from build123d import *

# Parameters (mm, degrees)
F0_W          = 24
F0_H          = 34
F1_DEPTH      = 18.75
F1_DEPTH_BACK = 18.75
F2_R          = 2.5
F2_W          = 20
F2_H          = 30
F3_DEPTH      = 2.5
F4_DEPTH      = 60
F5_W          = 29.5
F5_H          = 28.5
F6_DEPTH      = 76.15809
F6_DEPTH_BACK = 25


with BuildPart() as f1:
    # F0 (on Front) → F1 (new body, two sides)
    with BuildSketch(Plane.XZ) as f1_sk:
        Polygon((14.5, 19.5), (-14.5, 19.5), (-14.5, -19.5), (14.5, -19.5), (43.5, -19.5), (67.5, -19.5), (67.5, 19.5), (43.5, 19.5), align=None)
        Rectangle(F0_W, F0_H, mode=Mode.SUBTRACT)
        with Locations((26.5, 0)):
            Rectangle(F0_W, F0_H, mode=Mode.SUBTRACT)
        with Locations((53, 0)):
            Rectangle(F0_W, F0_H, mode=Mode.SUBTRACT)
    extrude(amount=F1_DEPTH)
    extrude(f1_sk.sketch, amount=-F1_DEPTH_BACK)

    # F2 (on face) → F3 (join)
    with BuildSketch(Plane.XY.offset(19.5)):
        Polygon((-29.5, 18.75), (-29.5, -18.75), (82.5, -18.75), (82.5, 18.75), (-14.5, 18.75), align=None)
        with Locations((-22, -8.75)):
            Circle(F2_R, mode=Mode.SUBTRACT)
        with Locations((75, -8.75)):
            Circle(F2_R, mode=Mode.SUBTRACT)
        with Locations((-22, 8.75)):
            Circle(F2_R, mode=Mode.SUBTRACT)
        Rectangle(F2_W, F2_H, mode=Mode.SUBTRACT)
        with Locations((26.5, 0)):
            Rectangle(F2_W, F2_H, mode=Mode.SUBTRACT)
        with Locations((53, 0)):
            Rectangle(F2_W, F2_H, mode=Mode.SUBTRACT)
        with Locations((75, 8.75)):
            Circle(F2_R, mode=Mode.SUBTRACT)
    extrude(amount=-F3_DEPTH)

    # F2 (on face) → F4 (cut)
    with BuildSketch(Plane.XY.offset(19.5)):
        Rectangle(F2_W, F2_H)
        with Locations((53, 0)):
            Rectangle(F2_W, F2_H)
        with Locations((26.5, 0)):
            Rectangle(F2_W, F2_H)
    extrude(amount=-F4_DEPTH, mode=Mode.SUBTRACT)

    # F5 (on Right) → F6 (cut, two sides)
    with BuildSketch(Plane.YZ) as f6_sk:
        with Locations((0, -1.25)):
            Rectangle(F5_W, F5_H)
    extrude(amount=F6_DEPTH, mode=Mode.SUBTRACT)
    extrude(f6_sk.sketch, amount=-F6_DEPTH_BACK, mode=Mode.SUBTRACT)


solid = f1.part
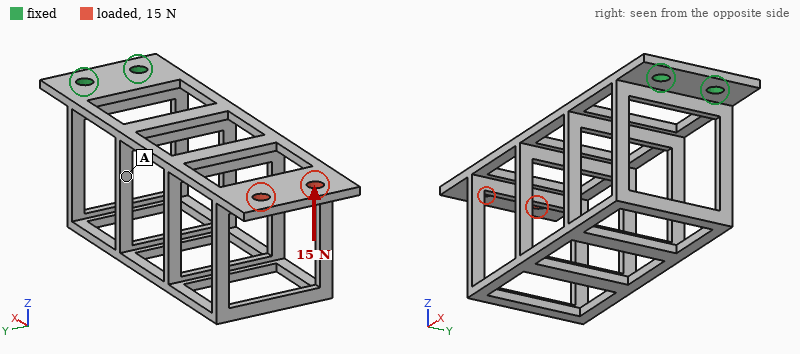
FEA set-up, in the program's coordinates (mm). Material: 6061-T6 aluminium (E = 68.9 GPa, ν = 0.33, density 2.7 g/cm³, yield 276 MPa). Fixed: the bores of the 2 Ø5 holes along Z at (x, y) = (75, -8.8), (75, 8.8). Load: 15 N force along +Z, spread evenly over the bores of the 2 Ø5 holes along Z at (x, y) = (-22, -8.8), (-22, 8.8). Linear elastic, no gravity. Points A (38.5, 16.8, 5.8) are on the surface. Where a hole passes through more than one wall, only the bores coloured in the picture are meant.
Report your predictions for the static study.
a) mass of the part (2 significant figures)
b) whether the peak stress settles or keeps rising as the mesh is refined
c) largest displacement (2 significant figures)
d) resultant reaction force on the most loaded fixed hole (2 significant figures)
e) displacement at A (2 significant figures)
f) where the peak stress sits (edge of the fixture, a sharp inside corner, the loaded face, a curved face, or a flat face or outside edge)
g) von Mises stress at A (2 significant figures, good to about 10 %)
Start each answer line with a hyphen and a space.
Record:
- 36 g
- keeps rising
- 1.2 mm
- 12 N
- 0.33 mm
- a sharp inside corner
- 9.0 MPa
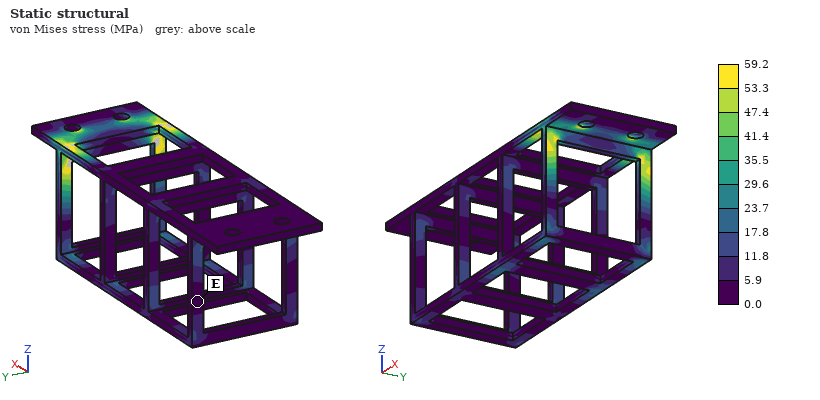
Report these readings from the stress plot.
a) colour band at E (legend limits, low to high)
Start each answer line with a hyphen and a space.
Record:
- 0.0 to 5.9 MPa
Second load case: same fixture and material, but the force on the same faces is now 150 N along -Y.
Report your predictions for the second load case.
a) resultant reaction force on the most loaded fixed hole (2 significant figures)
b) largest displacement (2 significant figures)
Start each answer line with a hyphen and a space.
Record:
- 630 N
- 0.61 mm
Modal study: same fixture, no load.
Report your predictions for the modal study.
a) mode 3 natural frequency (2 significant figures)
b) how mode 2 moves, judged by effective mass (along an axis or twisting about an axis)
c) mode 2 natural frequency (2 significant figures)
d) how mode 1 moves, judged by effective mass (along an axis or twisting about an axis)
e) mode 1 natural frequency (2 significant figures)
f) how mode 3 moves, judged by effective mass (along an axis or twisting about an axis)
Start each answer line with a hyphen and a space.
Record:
- 860 Hz
- along Y
- 570 Hz
- along Z
- 160 Hz
- along Y
